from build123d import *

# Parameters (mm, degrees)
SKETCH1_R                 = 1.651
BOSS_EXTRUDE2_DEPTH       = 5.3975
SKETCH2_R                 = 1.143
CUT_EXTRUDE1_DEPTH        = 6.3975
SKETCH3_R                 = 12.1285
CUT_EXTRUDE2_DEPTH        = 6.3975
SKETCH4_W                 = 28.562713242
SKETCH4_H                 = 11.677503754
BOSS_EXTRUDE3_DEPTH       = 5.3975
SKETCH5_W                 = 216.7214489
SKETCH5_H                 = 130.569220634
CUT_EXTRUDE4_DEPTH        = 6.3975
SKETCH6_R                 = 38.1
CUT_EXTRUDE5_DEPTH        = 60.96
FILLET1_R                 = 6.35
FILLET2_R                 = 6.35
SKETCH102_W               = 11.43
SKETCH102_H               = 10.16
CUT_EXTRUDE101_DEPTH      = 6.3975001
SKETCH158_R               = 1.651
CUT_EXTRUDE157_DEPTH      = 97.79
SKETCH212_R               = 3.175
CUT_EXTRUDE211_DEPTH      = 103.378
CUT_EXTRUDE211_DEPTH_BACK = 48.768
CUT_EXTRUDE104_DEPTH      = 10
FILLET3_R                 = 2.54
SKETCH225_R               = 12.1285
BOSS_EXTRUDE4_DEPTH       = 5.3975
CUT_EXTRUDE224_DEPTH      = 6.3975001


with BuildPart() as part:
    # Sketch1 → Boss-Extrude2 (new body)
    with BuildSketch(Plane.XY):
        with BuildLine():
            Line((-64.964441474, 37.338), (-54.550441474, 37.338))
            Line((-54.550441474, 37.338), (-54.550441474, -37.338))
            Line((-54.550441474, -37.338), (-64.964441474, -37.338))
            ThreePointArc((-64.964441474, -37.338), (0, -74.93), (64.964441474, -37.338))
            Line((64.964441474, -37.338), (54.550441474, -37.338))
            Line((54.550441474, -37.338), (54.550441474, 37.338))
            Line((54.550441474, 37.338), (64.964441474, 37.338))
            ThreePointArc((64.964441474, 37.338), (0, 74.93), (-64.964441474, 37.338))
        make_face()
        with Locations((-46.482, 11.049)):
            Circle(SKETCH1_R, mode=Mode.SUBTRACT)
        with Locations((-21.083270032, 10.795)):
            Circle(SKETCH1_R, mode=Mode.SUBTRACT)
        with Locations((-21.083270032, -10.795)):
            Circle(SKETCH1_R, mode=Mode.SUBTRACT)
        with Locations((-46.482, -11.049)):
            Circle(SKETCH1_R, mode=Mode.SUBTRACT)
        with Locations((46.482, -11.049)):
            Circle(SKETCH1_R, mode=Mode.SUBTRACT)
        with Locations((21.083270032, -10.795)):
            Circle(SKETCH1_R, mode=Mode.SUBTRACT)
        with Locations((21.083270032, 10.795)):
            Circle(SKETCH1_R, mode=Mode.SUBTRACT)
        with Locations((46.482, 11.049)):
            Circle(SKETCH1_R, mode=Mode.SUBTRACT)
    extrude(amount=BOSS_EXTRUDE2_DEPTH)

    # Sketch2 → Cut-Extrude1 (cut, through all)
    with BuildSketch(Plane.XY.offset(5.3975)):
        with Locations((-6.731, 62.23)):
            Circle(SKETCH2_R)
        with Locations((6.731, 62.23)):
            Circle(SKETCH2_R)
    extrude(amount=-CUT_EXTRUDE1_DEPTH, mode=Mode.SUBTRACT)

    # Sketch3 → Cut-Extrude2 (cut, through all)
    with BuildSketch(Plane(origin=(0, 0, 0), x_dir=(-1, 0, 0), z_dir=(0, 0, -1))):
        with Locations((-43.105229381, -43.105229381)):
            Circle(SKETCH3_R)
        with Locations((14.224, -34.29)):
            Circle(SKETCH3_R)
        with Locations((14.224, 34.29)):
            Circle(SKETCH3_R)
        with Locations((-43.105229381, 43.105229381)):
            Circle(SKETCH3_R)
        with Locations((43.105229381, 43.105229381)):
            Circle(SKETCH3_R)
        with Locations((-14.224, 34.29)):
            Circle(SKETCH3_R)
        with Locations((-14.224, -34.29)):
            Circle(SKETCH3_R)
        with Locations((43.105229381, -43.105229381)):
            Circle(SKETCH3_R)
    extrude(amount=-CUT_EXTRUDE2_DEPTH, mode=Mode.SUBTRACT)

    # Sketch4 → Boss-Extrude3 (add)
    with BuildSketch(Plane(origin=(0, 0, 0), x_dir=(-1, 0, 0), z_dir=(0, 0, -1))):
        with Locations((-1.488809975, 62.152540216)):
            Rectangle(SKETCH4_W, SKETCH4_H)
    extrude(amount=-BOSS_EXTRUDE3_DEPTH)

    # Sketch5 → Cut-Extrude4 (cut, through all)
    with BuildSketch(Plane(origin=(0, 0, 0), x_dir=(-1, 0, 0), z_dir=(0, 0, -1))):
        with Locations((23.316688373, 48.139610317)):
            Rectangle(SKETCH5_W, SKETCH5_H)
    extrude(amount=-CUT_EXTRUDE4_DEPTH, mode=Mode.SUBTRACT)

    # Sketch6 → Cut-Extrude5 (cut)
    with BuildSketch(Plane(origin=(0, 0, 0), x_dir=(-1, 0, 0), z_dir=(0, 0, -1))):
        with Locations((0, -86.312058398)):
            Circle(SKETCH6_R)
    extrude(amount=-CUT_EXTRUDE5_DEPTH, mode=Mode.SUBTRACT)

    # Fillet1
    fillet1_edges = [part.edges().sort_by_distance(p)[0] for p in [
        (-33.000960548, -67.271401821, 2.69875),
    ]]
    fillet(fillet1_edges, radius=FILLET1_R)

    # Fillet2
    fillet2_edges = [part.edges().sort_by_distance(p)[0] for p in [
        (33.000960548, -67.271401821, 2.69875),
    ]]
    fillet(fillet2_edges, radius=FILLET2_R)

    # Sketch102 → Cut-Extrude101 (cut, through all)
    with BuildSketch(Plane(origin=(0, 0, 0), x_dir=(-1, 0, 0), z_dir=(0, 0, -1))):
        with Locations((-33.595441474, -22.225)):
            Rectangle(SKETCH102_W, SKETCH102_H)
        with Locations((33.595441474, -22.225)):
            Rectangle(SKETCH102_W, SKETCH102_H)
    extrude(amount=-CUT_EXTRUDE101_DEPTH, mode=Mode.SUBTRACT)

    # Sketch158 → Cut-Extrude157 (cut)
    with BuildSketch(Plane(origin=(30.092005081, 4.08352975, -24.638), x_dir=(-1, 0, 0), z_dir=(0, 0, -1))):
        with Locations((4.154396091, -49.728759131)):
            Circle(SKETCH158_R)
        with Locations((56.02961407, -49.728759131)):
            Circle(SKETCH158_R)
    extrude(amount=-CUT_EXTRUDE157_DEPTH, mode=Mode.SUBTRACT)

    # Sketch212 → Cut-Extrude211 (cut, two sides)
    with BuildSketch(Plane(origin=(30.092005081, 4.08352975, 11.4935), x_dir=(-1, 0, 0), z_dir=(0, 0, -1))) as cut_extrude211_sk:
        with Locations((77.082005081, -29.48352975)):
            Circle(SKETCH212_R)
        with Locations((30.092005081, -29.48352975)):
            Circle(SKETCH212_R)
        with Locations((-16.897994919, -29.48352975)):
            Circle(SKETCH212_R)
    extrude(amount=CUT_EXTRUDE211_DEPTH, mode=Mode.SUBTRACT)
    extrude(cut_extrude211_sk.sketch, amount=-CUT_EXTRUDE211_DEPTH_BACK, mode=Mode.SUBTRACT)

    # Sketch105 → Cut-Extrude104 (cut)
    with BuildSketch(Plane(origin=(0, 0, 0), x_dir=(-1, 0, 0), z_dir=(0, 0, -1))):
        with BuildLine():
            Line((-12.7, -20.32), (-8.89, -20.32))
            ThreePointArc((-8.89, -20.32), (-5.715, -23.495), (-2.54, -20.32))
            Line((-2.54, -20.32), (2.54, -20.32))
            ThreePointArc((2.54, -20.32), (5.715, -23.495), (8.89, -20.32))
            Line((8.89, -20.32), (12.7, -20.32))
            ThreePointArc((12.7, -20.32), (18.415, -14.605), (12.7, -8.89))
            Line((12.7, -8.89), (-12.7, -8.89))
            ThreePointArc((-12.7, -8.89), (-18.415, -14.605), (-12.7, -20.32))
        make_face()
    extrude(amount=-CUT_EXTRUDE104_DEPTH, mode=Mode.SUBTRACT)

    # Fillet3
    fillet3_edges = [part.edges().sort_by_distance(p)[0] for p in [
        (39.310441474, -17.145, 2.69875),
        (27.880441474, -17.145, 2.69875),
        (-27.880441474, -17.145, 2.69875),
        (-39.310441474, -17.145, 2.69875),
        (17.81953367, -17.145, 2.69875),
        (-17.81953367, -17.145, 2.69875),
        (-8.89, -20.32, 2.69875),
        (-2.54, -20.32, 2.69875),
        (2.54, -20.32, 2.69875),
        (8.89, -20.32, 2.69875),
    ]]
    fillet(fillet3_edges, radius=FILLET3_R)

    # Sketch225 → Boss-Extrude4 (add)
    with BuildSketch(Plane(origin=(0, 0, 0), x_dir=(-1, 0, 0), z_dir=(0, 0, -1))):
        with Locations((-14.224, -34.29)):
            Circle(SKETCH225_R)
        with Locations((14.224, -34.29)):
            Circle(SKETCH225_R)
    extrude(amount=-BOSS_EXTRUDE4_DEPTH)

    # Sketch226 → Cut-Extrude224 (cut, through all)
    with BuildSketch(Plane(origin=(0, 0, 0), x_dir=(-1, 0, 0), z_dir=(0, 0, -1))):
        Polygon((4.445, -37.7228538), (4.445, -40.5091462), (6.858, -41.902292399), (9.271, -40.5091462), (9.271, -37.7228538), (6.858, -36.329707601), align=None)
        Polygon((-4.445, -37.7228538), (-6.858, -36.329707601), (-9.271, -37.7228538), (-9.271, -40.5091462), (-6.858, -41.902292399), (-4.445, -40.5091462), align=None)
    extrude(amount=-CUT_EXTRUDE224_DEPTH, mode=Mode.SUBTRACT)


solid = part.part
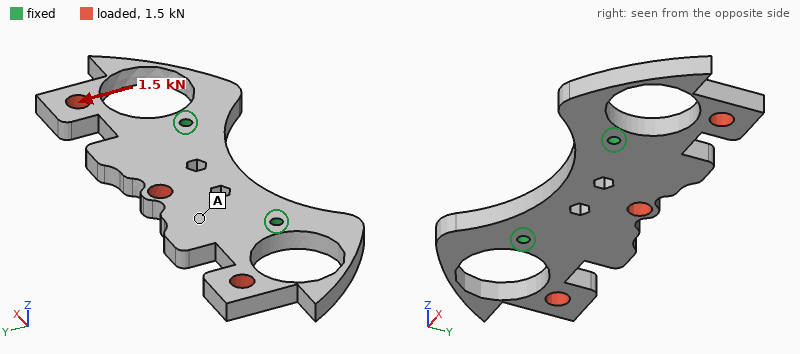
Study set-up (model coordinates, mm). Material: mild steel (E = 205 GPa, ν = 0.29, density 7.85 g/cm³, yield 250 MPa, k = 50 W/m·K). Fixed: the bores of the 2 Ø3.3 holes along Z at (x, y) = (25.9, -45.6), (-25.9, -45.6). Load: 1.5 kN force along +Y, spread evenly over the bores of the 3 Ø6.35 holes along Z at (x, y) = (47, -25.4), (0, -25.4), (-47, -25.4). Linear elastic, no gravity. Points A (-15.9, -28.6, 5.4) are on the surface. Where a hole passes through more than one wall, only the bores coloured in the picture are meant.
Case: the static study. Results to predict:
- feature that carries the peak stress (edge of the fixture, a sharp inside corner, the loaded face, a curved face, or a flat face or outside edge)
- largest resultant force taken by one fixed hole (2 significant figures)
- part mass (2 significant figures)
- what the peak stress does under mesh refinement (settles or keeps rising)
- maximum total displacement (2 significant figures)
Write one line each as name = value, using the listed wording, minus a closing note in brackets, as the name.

feature that carries the peak stress = a sharp inside corner
largest resultant force taken by one fixed hole = 770 N
part mass = 130 g
what the peak stress does under mesh refinement = keeps rising
maximum total displacement = 35 µm
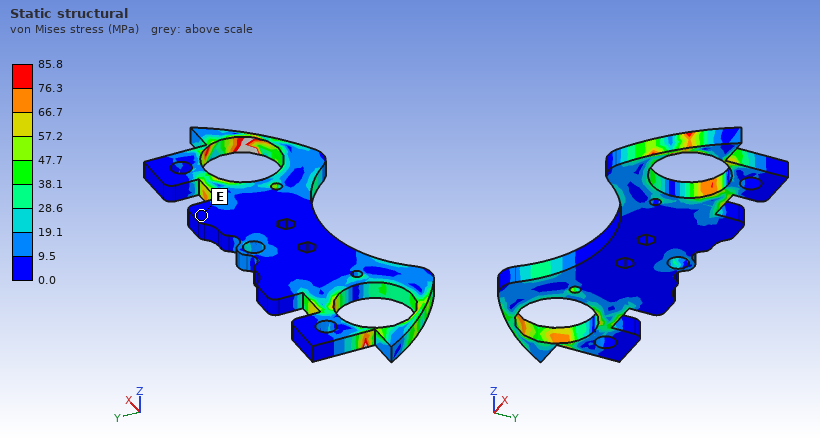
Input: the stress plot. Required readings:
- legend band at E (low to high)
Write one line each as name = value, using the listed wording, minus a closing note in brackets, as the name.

legend band at E = 0.0 to 9.5 MPa
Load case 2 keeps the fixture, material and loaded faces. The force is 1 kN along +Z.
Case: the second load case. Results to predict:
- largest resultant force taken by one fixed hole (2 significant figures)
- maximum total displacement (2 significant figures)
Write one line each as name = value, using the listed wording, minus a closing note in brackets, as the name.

largest resultant force taken by one fixed hole = 500 N
maximum total displacement = 0.14 mm
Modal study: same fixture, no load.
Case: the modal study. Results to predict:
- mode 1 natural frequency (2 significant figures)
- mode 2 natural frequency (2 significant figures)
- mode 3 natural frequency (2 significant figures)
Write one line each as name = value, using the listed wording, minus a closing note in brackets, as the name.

mode 1 natural frequency = 2700 Hz
mode 2 natural frequency = 2800 Hz
mode 3 natural frequency = 4000 Hz
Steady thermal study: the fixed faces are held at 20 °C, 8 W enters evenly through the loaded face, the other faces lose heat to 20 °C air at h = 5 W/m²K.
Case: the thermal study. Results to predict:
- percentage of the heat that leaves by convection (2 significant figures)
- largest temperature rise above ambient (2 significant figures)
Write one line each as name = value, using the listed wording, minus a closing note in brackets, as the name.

percentage of the heat that leaves by convection = 6.5 %
largest temperature rise above ambient = 32 K
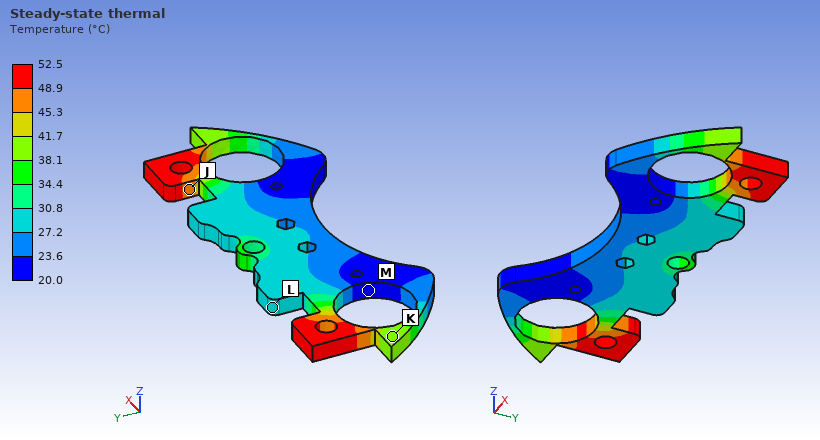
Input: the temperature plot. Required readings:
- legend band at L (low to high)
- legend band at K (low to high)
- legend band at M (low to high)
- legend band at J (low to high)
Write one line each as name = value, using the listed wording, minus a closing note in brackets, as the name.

legend band at L = 27.2 to 30.8 °C
legend band at K = 38.1 to 41.7 °C
legend band at M = 20.0 to 23.6 °C
legend band at J = 45.3 to 48.9 °C
